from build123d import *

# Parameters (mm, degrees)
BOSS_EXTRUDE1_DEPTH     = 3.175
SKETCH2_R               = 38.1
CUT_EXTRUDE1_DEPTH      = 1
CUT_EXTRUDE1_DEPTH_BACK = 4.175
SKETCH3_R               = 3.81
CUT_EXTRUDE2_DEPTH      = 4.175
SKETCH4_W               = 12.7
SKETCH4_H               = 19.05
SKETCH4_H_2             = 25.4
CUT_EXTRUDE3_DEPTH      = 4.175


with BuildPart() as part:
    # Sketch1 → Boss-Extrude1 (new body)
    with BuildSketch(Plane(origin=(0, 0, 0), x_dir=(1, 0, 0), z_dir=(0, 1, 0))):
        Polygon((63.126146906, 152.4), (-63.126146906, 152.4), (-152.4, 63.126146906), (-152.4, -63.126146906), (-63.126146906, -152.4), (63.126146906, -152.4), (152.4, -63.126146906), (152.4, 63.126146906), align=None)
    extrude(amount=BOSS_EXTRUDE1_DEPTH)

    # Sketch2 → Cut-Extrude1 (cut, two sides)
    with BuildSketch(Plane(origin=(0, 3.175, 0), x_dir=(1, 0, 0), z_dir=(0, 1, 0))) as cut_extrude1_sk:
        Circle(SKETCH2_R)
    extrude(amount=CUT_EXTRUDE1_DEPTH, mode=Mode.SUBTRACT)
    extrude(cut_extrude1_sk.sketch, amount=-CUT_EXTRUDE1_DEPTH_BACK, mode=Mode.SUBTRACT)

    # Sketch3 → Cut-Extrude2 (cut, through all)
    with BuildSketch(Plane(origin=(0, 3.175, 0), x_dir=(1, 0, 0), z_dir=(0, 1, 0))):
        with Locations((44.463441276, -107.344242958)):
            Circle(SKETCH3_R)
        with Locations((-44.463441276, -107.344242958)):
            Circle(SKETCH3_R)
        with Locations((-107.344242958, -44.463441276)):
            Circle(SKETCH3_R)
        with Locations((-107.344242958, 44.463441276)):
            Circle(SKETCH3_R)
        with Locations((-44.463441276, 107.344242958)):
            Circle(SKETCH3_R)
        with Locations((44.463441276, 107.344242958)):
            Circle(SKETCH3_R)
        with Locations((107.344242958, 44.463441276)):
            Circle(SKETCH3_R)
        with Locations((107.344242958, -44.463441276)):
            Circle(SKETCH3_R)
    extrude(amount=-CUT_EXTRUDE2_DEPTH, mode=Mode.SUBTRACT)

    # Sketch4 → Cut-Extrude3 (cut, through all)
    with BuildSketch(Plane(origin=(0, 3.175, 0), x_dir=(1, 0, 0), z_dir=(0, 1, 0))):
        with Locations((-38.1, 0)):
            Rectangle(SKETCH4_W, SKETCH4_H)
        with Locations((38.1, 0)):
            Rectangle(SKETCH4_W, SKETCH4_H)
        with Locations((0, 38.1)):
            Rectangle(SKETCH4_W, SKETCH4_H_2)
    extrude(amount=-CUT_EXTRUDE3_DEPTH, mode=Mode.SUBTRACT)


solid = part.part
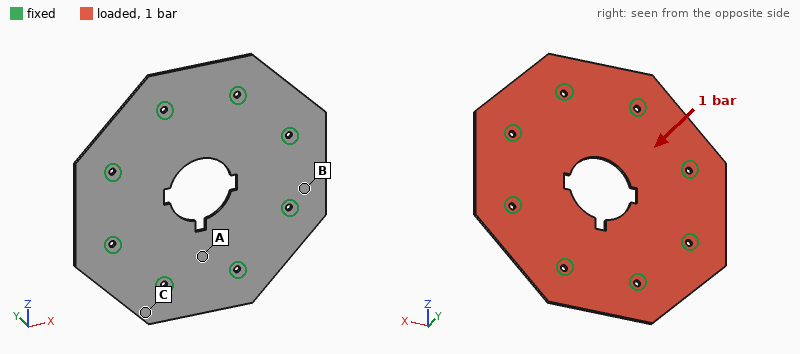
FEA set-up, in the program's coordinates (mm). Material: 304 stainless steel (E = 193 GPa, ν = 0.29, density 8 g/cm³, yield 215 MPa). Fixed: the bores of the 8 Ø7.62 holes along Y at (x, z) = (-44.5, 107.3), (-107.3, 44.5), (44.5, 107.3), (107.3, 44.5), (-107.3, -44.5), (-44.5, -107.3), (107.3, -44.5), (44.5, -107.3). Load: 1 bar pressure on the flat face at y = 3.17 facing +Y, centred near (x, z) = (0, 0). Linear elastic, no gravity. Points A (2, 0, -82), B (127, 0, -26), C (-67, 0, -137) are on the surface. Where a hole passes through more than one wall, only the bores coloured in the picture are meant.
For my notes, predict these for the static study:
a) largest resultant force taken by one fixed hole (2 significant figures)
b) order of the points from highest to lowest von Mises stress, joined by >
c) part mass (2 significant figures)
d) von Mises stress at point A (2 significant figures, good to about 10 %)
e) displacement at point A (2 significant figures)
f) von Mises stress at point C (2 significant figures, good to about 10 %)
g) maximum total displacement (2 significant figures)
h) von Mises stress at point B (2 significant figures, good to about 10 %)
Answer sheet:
900 N
A > B > C
1.8 kg
46 MPa
0.15 mm
12 MPa
0.43 mm
26 MPa
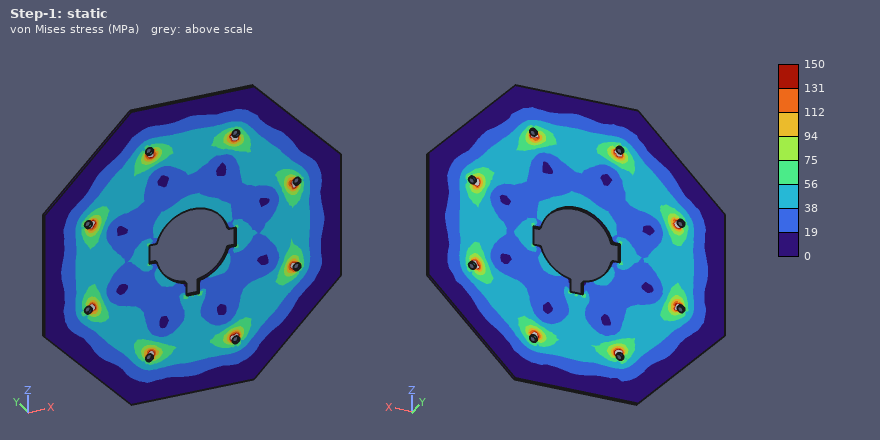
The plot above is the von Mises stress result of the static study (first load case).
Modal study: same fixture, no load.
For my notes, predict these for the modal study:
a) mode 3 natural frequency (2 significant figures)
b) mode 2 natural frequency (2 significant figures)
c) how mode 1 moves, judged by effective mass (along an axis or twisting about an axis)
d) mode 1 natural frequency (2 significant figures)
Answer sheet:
910 Hz
910 Hz
along Y
580 Hz
